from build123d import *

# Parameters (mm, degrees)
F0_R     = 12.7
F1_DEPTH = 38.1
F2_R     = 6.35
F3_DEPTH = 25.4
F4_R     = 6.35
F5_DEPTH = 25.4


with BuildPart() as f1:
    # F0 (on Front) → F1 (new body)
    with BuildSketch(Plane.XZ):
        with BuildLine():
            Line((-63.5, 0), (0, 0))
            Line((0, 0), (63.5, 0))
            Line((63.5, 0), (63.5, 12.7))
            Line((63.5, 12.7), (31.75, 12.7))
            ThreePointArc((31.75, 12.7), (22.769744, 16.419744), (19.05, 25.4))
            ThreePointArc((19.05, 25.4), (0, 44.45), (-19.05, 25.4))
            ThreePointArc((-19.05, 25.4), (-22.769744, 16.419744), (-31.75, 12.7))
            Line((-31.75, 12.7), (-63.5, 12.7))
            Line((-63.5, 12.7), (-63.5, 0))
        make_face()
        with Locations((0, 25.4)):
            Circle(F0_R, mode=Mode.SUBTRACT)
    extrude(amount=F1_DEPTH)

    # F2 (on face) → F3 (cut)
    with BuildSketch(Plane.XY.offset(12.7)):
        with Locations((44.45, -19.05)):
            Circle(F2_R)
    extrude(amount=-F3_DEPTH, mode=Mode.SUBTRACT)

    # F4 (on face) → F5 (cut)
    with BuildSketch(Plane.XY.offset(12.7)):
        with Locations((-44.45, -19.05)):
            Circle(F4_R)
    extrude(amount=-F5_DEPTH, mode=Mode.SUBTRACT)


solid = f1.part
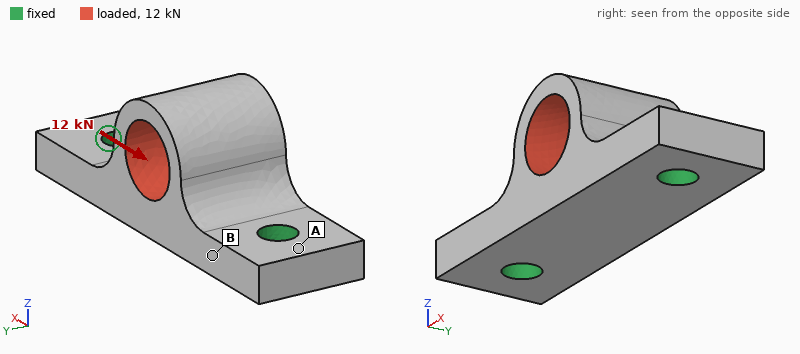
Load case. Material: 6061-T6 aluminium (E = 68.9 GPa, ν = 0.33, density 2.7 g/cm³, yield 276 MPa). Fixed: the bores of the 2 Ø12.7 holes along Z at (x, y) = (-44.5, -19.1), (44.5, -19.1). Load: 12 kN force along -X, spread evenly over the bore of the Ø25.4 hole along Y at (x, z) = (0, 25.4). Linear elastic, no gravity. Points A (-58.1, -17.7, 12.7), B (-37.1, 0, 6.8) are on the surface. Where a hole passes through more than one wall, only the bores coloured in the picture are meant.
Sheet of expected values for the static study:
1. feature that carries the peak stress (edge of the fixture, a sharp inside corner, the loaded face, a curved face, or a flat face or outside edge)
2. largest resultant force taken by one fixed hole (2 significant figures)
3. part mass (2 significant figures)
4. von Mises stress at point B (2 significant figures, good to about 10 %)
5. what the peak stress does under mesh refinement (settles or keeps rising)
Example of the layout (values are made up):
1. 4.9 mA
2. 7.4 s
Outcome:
1. edge of the fixture
2. 6.8 kN
3. 220 g
4. 12 MPa
5. keeps rising
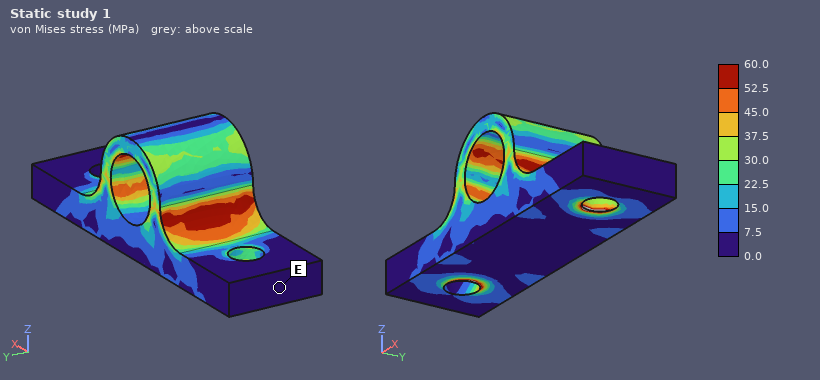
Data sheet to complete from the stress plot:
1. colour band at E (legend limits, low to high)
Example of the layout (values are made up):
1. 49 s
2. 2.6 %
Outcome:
1. 0.0 to 7.5 MPa
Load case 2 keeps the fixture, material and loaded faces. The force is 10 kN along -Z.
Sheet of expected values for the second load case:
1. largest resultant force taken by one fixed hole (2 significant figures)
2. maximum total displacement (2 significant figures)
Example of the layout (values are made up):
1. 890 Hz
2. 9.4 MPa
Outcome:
1. 5.3 kN
2. 43 µm
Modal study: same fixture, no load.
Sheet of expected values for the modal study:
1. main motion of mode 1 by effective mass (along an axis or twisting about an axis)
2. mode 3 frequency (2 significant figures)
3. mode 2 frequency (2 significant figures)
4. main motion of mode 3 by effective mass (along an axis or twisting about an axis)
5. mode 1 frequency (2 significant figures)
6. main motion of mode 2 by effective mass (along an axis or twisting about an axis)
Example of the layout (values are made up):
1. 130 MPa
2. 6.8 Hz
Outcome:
1. along Y
2. 10 kHz
3. 7400 Hz
4. along X
5. 5300 Hz
6. along Z
